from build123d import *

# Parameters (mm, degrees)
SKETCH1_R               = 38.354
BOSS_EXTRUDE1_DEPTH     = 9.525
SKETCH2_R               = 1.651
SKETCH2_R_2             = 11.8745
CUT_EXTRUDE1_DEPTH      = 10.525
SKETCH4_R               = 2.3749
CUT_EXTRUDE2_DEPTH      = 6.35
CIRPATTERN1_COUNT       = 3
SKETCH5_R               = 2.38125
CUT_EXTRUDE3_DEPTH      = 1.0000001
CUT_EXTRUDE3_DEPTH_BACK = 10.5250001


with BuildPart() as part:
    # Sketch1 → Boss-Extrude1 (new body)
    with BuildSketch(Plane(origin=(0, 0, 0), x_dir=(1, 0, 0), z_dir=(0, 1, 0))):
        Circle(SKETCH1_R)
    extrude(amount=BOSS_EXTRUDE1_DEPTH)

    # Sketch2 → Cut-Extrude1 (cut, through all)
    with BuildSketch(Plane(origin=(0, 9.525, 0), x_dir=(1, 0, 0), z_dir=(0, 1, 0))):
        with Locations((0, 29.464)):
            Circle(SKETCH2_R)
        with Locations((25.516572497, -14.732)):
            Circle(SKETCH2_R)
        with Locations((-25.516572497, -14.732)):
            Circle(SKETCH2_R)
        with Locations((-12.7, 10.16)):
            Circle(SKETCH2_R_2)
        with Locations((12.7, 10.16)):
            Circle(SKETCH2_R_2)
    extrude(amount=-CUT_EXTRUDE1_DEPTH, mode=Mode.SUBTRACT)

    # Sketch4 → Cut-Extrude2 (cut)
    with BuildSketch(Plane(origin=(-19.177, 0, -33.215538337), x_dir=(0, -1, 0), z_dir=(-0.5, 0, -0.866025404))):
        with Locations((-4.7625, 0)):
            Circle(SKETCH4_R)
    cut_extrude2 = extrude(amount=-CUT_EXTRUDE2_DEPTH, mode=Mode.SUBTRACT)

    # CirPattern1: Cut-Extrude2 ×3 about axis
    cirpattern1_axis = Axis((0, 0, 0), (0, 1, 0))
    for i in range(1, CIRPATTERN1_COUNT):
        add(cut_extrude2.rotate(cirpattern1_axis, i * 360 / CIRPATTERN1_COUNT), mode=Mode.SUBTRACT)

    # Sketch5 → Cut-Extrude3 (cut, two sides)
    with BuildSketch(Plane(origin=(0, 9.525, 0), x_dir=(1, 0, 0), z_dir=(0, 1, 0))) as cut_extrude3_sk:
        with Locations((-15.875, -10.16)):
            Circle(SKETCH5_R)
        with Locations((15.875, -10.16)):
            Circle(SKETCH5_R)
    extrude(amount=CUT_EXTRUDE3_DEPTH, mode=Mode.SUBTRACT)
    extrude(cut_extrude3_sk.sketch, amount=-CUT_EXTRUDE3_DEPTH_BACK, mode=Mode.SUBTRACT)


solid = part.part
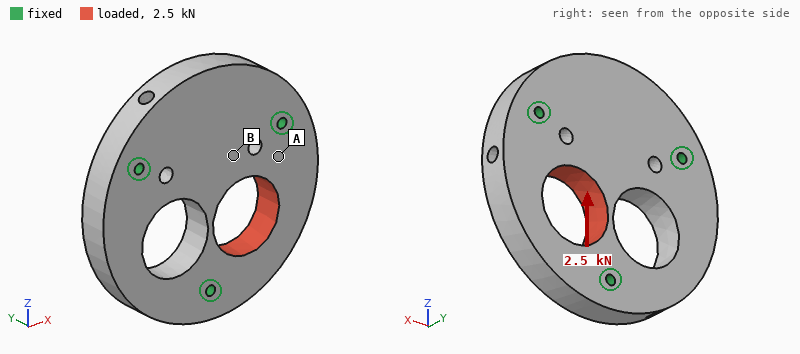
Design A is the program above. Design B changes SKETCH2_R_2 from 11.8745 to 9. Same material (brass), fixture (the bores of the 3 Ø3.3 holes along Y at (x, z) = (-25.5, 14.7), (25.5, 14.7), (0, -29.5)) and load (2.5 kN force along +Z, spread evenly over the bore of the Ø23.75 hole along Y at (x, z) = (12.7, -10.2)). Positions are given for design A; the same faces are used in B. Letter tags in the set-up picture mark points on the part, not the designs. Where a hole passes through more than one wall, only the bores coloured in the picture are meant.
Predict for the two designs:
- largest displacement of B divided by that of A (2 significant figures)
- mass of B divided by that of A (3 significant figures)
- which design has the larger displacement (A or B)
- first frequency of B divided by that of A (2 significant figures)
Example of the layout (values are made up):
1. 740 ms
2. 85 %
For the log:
1. 0.78
2. 1.10
3. A
4. 1.0
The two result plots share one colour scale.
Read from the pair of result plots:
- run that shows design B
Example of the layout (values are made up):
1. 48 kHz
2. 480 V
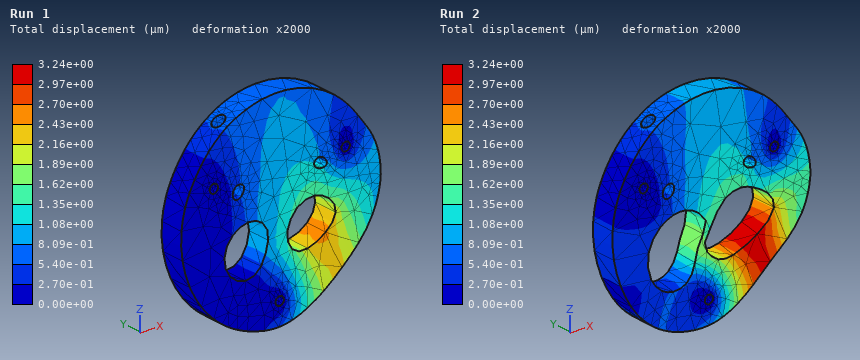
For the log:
1. Run 1
